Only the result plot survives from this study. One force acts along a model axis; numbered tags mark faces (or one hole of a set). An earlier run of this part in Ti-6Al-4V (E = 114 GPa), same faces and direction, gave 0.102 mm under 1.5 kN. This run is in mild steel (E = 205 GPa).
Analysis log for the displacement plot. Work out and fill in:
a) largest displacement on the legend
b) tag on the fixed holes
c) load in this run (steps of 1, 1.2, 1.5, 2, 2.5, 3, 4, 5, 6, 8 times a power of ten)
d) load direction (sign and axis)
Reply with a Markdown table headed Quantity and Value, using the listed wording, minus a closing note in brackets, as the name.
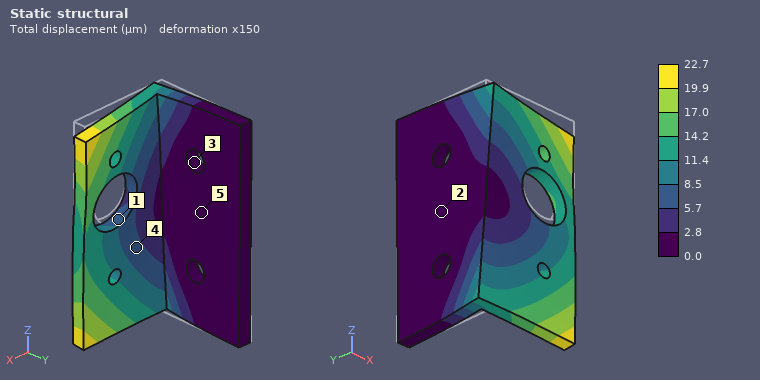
| Quantity | Value |
|---|---|
| largest displacement on the legend | 22.7 µm |
| tag on the fixed holes | 3 |
| load in this run | 600 N |
| load direction | -Z |
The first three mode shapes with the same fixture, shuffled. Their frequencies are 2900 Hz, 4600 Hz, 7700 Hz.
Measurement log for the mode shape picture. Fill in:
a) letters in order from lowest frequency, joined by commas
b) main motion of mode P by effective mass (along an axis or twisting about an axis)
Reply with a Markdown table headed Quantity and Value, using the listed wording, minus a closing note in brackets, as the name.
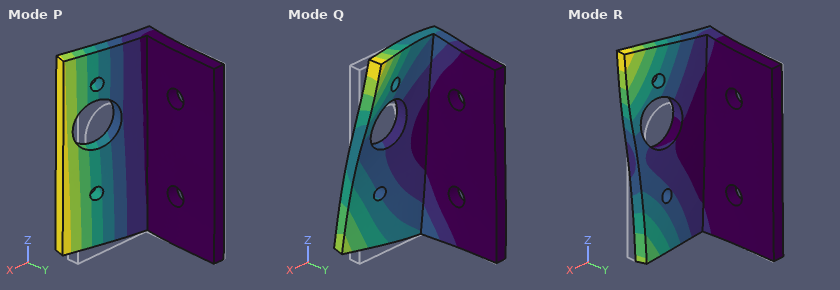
| Quantity | Value |
|---|---|
| letters in order from lowest frequency, joined by commas | P, R, Q |
| main motion of mode P by effective mass | along Y |
